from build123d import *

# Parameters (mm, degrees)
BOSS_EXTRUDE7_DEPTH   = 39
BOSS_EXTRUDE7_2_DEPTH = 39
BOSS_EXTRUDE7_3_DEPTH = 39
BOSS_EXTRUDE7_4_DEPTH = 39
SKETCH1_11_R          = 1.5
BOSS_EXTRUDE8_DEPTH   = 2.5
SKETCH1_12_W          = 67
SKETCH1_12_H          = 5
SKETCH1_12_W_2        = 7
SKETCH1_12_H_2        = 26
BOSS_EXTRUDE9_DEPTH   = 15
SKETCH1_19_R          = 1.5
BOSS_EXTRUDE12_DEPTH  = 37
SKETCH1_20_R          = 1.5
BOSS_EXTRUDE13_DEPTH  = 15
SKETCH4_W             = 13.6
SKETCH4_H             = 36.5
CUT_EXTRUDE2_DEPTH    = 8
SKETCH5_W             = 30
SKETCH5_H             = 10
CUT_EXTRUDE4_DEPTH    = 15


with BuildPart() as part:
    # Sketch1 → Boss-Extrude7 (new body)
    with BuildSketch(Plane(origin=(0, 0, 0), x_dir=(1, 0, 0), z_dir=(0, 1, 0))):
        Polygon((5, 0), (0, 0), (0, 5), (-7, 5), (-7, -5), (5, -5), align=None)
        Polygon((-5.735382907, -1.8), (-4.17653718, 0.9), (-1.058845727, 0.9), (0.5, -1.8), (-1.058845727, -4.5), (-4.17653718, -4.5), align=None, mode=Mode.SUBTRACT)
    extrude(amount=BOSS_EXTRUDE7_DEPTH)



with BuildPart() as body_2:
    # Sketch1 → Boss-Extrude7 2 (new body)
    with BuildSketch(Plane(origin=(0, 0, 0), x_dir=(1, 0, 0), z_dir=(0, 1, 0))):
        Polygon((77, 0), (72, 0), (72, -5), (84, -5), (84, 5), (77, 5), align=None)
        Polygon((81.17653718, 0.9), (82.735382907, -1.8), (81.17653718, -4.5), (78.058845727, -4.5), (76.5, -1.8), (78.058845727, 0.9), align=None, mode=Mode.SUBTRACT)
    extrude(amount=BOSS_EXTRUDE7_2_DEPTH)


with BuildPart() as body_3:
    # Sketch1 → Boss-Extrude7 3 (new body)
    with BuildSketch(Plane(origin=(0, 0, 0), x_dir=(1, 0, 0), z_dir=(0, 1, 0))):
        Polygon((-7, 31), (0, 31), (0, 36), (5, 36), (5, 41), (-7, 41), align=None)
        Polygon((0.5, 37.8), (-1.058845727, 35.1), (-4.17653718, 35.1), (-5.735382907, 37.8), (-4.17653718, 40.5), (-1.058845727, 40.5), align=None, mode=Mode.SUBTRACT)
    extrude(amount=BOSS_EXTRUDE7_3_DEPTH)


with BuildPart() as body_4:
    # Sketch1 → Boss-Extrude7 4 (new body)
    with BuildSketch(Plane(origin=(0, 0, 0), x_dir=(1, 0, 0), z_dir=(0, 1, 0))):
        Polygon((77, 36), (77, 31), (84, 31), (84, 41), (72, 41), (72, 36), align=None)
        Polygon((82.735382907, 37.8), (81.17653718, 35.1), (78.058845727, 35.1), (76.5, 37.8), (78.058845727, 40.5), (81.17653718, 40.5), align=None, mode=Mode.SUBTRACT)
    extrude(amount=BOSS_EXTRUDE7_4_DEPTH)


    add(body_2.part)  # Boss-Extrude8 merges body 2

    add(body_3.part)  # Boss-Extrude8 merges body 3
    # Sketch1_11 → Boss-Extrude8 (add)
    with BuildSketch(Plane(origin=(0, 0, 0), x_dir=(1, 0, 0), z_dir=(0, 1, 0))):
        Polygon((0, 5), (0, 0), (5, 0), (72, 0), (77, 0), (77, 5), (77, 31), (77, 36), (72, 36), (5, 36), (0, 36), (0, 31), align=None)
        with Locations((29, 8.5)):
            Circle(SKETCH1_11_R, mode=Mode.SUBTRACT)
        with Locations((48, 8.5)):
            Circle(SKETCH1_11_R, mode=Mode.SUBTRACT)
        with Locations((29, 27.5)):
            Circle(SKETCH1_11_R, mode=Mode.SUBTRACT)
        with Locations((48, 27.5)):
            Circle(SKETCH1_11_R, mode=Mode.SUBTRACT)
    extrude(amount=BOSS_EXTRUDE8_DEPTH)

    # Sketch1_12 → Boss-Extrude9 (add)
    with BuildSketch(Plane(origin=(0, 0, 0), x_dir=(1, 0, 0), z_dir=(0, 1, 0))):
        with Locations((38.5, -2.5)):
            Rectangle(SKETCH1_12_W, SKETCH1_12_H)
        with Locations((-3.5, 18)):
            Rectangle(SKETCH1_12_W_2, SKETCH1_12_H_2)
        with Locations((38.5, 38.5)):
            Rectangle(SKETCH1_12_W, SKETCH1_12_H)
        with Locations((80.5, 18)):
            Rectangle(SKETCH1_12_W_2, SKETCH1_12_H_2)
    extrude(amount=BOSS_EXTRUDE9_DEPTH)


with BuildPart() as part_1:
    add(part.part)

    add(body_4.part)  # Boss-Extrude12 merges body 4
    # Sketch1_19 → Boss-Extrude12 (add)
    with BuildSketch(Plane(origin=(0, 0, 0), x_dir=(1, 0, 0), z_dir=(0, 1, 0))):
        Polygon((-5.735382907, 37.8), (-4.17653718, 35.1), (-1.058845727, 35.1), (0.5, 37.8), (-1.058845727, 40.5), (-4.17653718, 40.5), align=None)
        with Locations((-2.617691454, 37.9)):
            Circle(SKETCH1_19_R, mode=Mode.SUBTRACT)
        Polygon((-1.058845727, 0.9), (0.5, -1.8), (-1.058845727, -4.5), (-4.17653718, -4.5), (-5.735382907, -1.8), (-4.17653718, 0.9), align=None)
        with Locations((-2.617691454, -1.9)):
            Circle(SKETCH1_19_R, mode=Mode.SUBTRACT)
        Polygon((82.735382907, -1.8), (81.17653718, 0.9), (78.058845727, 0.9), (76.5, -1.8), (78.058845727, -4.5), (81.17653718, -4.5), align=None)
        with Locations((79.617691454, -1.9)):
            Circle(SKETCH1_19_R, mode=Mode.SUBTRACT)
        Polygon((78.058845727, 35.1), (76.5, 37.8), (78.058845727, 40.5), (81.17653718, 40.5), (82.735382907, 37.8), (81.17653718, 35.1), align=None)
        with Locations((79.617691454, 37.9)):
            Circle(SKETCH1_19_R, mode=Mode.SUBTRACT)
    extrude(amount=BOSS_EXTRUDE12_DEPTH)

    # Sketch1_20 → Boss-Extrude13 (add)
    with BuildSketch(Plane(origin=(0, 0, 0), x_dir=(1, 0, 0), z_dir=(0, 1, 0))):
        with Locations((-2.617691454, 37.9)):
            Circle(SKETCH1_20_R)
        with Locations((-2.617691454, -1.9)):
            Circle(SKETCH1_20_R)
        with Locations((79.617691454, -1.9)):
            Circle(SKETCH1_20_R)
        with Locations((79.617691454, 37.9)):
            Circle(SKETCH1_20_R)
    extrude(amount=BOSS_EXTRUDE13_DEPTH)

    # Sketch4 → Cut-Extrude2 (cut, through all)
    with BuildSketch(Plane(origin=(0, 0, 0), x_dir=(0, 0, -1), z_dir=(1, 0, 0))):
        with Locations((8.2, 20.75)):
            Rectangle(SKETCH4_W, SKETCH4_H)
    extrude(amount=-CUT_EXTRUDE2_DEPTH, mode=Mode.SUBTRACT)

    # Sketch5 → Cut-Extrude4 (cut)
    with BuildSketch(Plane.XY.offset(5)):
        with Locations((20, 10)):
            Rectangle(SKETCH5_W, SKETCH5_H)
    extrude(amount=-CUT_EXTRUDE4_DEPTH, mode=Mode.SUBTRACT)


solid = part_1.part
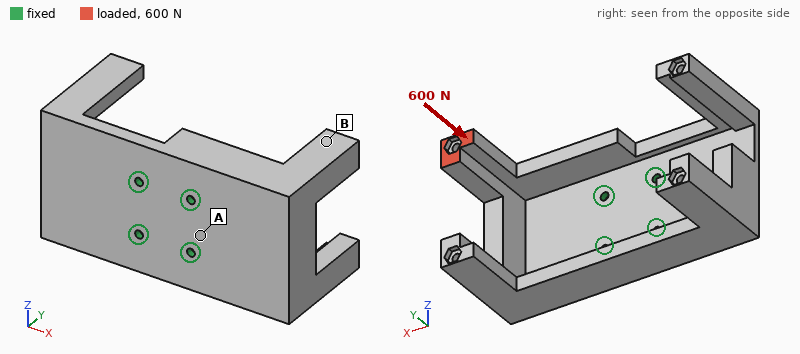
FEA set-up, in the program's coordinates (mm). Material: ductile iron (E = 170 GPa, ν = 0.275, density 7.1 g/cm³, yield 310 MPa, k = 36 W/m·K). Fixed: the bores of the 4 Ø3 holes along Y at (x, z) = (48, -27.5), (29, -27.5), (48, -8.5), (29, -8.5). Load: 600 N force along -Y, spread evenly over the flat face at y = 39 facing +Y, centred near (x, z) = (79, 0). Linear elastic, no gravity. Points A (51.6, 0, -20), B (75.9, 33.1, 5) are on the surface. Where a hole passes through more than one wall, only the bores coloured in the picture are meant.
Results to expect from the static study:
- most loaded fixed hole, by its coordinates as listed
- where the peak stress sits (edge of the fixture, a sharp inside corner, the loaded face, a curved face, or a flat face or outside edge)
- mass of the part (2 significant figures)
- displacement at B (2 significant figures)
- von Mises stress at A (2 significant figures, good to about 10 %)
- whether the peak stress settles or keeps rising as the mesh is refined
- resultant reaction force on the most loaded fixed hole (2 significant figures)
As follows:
(48, -8.5)
edge of the fixture
230 g
0.18 mm
55 MPa
keeps rising
1.1 kN
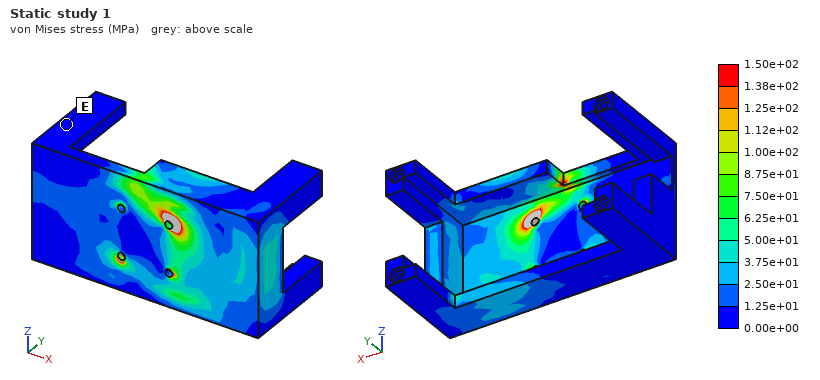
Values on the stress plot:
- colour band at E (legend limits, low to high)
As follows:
0.00e+00 to 1.25e+01 MPa
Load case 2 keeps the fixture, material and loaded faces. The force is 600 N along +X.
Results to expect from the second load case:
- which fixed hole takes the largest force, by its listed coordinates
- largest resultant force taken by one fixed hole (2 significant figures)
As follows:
(29, -8.5)
890 N
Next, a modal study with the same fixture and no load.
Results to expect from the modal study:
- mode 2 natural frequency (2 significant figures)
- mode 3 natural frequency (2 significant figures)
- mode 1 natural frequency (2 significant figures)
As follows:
1200 Hz
1400 Hz
1000 Hz
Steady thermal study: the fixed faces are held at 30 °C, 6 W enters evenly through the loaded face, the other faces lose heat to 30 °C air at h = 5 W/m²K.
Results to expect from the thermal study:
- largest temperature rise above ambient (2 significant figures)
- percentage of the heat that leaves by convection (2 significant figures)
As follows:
83 K
19 %
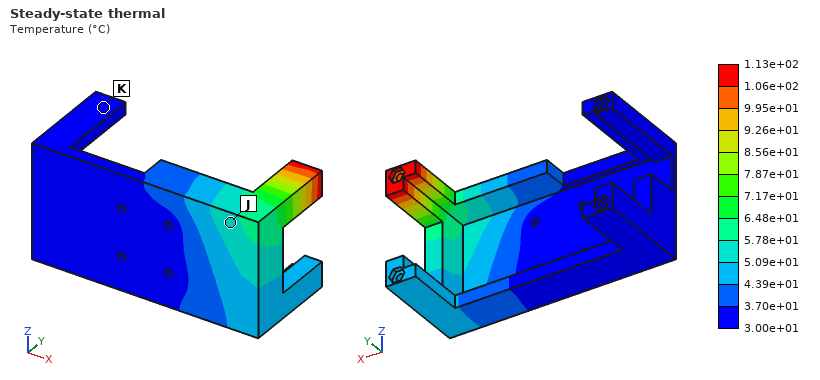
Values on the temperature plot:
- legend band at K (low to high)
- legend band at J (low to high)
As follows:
3.00e+01 to 3.70e+01 °C
5.09e+01 to 5.78e+01 °C
